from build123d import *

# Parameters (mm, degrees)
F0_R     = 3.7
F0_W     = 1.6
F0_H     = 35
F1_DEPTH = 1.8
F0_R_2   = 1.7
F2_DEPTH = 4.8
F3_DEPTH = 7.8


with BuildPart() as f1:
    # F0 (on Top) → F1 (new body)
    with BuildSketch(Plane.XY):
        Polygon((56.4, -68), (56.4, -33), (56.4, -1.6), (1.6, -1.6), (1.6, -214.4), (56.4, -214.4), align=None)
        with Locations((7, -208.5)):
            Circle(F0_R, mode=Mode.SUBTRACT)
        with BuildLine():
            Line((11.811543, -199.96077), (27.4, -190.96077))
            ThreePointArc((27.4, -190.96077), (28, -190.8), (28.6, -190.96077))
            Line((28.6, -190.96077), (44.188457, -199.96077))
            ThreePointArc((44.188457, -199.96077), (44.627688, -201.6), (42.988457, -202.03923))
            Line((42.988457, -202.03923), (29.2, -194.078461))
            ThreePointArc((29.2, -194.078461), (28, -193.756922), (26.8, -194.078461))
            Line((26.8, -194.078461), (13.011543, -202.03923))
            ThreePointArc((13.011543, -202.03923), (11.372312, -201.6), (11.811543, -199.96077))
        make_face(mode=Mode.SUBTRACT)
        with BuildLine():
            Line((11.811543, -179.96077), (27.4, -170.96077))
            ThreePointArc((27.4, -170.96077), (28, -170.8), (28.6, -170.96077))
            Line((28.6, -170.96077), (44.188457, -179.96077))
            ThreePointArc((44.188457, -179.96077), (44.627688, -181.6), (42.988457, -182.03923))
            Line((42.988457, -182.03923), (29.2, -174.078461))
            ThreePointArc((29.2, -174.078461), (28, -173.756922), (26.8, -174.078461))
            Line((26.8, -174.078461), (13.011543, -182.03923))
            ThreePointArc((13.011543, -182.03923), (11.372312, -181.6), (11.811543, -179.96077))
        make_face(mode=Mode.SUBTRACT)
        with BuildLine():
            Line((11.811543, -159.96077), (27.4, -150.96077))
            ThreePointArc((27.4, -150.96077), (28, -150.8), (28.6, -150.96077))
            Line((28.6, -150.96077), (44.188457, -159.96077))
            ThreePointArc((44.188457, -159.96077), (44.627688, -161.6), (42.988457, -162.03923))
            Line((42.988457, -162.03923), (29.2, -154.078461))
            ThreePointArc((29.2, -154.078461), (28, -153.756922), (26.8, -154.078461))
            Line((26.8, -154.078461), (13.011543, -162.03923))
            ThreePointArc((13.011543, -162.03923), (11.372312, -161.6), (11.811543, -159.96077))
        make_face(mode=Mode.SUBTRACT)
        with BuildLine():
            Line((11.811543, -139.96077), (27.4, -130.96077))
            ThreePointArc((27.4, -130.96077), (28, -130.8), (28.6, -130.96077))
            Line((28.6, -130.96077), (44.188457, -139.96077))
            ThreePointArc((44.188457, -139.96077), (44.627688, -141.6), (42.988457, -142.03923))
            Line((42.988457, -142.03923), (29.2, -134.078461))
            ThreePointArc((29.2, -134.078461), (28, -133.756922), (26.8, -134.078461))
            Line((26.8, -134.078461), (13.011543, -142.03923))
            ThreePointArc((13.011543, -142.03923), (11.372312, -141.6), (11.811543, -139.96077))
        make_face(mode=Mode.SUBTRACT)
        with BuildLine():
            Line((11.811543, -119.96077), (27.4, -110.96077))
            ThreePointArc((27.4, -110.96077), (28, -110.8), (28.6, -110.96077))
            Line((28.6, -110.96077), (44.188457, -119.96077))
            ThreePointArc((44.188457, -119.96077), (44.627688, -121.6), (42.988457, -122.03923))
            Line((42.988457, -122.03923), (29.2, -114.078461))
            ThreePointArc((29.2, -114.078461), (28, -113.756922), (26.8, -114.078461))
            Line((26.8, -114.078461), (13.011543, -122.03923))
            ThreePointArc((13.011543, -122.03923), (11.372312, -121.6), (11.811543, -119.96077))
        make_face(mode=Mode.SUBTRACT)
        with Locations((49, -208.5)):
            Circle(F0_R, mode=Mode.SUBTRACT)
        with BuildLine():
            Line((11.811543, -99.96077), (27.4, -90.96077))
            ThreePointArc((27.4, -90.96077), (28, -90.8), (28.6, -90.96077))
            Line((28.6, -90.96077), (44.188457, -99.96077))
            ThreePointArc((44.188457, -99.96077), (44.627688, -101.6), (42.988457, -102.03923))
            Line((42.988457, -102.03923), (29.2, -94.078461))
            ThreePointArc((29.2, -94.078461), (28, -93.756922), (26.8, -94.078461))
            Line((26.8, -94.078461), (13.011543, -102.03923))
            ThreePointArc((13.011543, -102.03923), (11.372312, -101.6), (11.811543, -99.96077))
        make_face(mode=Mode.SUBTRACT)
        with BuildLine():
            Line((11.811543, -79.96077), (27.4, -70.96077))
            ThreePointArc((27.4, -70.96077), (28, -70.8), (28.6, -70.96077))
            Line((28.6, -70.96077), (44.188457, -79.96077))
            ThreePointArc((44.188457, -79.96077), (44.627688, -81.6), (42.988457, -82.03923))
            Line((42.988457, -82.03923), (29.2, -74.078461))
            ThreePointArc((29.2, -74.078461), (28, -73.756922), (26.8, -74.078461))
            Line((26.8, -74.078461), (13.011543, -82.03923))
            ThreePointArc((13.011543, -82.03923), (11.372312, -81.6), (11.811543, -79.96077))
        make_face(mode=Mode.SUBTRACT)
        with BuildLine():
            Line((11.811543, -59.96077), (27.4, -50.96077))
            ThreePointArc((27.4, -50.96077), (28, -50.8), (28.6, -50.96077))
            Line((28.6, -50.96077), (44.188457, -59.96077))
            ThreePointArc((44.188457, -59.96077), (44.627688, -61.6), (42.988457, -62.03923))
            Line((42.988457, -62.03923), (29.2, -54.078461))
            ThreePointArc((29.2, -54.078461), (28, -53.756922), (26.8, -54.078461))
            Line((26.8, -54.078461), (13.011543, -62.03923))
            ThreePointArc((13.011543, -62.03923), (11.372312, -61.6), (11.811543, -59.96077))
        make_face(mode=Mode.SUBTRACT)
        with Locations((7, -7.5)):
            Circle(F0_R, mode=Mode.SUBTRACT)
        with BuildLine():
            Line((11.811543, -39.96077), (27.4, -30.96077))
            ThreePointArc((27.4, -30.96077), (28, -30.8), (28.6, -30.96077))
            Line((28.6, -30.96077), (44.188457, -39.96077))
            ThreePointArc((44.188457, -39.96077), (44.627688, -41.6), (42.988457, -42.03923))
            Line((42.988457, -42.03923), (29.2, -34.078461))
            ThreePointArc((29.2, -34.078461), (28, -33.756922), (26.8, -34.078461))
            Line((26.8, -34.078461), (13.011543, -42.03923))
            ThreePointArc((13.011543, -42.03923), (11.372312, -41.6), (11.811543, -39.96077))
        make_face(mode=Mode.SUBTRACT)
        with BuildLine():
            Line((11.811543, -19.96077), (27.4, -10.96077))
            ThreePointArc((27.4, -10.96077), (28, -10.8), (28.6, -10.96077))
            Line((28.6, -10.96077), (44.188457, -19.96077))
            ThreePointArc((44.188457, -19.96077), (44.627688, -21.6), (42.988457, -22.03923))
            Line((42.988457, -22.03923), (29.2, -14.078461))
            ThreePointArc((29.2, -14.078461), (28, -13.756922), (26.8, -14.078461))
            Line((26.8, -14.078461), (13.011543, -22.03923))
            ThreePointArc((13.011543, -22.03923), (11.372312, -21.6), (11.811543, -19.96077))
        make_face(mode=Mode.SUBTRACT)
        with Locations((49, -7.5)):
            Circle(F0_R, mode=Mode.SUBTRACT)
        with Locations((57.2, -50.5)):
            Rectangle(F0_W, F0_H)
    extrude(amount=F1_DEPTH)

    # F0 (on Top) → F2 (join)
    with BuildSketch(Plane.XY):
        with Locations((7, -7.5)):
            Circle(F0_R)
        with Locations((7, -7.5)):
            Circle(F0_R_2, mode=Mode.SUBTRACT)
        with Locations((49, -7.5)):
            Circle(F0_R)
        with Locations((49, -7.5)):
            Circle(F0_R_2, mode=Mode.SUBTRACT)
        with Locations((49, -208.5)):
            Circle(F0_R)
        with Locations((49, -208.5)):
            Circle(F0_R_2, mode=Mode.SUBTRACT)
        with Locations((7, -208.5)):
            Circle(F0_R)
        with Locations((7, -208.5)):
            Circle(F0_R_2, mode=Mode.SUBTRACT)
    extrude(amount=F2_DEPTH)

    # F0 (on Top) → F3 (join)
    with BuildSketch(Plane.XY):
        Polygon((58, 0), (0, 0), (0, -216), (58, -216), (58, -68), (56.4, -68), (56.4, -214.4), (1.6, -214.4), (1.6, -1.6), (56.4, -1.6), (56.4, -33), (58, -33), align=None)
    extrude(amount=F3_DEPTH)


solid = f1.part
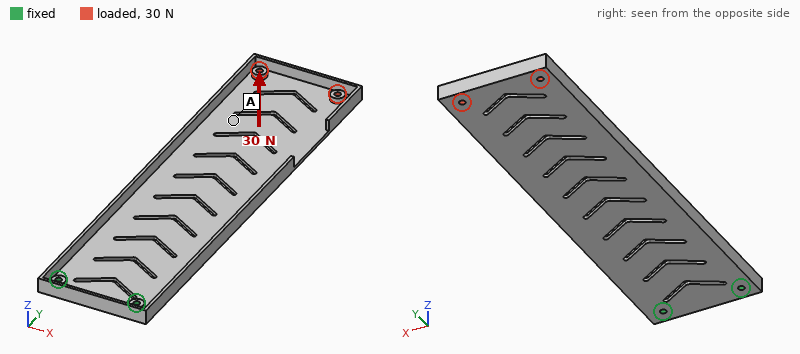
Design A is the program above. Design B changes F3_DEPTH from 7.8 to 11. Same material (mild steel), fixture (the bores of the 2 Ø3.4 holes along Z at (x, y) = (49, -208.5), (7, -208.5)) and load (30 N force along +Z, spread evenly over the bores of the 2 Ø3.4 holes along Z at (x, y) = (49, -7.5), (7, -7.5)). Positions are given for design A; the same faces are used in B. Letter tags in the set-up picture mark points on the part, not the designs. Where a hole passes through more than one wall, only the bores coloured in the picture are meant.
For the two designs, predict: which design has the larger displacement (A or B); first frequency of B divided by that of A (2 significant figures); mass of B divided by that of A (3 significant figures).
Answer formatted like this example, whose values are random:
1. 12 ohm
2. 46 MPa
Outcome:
1. A
2. 1.3
3. 1.10
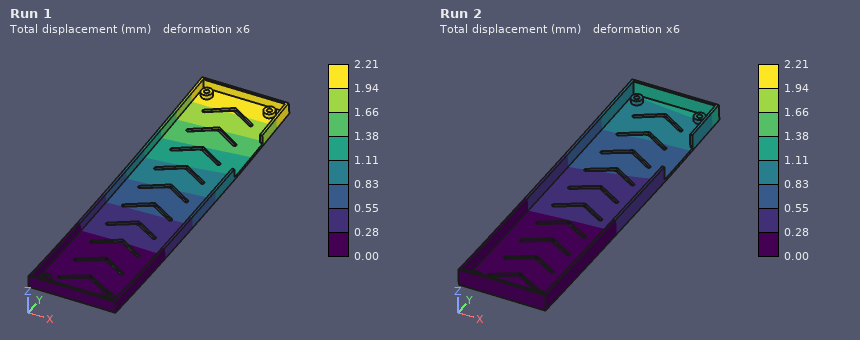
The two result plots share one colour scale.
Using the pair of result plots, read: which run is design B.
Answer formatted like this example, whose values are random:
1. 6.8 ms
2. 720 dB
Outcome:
1. Run 2
